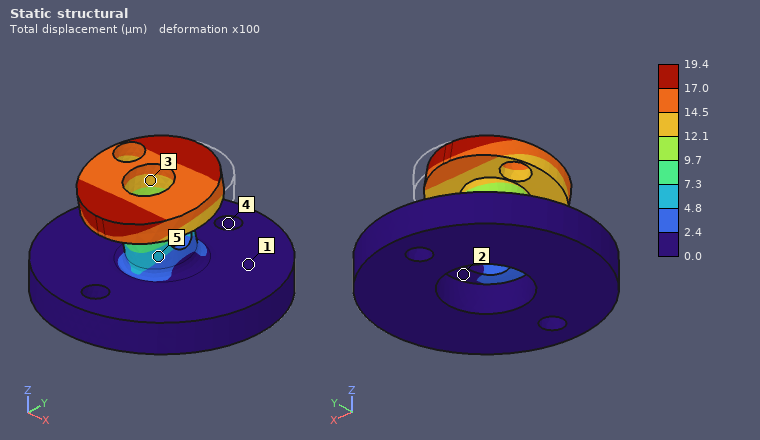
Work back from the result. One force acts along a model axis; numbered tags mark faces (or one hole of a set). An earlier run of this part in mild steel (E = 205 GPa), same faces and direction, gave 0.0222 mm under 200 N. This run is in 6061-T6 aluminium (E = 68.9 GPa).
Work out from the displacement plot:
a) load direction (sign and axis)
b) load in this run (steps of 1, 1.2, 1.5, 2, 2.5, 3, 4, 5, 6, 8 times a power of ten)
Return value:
-Y
60 N
